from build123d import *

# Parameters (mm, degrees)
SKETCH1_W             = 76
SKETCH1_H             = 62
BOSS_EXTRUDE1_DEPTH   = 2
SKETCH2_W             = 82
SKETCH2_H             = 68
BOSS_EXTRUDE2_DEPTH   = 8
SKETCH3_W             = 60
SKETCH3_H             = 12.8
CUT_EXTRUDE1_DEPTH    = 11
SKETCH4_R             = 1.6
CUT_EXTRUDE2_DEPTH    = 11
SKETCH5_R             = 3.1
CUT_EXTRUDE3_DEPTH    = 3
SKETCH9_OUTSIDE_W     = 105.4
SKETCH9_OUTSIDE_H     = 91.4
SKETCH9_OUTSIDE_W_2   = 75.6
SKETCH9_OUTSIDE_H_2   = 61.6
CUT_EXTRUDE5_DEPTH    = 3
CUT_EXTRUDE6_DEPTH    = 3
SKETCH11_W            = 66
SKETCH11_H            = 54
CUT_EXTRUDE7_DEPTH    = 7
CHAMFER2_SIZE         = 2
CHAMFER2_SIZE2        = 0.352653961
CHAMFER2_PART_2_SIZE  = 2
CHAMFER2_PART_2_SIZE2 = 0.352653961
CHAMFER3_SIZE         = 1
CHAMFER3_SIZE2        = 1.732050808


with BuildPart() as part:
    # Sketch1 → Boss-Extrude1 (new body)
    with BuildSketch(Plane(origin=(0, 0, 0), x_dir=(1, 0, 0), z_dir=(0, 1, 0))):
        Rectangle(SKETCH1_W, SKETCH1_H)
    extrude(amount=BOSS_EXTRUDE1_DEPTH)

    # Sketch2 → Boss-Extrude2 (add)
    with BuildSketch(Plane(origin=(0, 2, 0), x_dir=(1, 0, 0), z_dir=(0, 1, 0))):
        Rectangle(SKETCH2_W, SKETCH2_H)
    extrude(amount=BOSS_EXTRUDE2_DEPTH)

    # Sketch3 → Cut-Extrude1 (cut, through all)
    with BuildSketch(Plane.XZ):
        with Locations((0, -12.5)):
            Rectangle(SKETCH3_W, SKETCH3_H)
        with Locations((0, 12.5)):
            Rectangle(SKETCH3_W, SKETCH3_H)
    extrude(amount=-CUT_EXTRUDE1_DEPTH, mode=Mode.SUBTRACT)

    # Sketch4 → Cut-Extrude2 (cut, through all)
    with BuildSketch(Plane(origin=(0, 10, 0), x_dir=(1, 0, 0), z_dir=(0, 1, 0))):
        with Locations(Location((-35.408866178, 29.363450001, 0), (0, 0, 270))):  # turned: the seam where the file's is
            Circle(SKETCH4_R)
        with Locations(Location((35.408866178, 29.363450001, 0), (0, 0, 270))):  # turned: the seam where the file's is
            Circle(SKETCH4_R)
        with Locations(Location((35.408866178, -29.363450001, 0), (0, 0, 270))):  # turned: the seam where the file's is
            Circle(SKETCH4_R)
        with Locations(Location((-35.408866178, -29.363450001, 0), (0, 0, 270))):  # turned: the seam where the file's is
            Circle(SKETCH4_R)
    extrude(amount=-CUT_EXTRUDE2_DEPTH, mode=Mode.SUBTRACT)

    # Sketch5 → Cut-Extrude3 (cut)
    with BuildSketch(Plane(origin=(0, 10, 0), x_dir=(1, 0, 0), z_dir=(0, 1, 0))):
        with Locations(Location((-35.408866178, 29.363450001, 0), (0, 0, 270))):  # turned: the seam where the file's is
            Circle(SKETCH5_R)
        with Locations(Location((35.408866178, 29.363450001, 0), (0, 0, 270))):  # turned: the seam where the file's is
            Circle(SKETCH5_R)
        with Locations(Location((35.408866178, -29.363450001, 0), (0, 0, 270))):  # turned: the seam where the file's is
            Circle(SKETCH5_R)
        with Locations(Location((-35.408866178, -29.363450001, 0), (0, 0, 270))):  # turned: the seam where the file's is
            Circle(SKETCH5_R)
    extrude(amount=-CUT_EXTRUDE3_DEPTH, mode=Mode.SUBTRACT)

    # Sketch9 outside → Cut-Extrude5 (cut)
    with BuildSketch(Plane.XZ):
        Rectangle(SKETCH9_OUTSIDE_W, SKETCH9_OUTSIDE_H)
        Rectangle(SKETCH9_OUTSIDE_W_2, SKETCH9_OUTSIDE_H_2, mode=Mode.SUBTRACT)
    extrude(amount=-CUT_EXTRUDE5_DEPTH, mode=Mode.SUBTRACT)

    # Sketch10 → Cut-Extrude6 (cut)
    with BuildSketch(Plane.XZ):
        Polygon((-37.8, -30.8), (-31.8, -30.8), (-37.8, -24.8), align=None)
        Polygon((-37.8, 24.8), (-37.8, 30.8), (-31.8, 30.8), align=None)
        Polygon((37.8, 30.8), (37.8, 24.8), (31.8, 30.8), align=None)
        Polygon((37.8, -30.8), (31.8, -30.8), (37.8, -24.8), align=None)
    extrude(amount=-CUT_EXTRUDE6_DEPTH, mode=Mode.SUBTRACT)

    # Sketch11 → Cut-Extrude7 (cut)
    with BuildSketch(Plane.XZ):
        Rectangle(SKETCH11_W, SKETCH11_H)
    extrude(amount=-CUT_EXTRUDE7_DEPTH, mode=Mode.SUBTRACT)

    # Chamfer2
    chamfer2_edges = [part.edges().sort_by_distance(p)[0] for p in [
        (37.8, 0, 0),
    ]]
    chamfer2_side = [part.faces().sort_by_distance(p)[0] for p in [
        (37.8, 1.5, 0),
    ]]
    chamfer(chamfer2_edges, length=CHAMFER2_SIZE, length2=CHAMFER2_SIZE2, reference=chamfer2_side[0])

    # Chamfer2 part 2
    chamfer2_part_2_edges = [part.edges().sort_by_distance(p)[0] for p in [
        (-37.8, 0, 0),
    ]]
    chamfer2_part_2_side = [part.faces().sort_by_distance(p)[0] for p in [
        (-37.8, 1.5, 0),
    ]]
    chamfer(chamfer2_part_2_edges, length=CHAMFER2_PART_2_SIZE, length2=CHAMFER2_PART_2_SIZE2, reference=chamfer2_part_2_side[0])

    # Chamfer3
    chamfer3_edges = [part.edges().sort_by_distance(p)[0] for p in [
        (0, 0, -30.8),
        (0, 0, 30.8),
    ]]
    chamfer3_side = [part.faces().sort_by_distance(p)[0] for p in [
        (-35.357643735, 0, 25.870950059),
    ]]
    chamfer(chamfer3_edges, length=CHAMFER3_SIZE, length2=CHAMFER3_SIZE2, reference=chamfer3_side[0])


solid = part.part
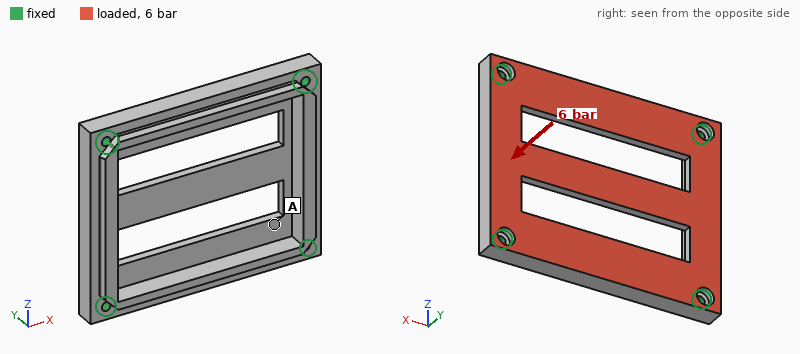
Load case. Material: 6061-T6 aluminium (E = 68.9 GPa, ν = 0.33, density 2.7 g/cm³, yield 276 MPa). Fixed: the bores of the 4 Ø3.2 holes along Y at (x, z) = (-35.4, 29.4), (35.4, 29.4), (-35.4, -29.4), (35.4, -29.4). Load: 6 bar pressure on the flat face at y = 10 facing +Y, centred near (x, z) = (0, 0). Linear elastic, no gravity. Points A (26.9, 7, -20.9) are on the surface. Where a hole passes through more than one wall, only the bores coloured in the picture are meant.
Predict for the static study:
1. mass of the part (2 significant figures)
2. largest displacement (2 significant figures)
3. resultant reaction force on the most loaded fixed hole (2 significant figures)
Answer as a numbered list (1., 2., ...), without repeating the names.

1. 61 g
2. 0.28 mm
3. 670 N
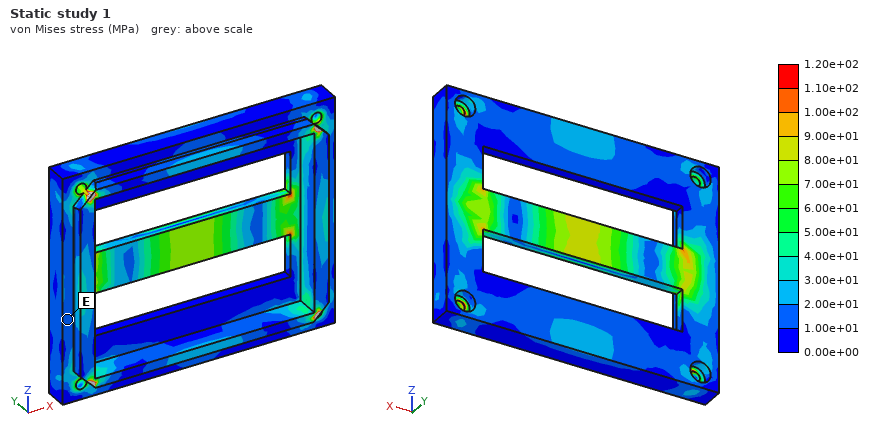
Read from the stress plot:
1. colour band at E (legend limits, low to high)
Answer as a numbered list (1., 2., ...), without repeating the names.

1. 1.00e+01 to 2.00e+01 MPa
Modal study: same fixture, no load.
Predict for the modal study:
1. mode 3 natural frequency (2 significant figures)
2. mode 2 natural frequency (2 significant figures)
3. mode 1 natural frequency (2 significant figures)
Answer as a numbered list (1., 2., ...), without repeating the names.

1. 6600 Hz
2. 6500 Hz
3. 3100 Hz
